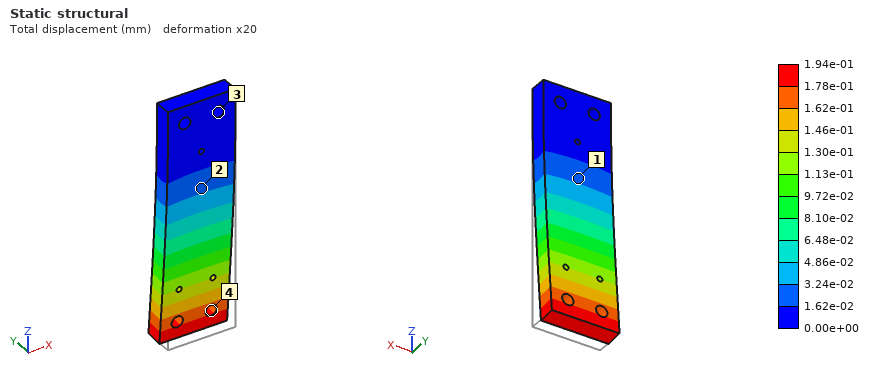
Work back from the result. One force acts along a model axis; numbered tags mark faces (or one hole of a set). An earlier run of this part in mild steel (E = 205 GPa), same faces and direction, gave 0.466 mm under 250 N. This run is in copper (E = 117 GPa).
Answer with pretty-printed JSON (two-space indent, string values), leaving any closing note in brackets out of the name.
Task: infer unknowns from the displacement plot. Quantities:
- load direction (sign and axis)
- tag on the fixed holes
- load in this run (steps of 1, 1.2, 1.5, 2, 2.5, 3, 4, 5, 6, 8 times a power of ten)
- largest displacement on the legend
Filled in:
{
  "load direction": "+Y",
  "tag on the fixed holes": "3",
  "load in this run": "60 N",
  "largest displacement on the legend": "1.94e-01 mm"
}
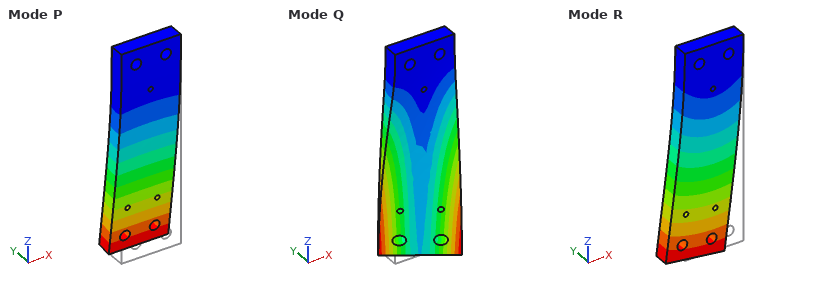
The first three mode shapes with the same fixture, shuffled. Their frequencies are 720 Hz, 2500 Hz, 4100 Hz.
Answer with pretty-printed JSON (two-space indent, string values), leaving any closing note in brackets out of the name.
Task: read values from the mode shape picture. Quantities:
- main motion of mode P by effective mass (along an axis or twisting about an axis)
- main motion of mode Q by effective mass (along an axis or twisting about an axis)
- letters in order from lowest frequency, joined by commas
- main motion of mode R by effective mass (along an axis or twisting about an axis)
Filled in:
{
  "main motion of mode P by effective mass": "along Y",
  "main motion of mode Q by effective mass": "twisting about Z",
  "letters in order from lowest frequency, joined by commas": "P, R, Q",
  "main motion of mode R by effective mass": "along X"
}
